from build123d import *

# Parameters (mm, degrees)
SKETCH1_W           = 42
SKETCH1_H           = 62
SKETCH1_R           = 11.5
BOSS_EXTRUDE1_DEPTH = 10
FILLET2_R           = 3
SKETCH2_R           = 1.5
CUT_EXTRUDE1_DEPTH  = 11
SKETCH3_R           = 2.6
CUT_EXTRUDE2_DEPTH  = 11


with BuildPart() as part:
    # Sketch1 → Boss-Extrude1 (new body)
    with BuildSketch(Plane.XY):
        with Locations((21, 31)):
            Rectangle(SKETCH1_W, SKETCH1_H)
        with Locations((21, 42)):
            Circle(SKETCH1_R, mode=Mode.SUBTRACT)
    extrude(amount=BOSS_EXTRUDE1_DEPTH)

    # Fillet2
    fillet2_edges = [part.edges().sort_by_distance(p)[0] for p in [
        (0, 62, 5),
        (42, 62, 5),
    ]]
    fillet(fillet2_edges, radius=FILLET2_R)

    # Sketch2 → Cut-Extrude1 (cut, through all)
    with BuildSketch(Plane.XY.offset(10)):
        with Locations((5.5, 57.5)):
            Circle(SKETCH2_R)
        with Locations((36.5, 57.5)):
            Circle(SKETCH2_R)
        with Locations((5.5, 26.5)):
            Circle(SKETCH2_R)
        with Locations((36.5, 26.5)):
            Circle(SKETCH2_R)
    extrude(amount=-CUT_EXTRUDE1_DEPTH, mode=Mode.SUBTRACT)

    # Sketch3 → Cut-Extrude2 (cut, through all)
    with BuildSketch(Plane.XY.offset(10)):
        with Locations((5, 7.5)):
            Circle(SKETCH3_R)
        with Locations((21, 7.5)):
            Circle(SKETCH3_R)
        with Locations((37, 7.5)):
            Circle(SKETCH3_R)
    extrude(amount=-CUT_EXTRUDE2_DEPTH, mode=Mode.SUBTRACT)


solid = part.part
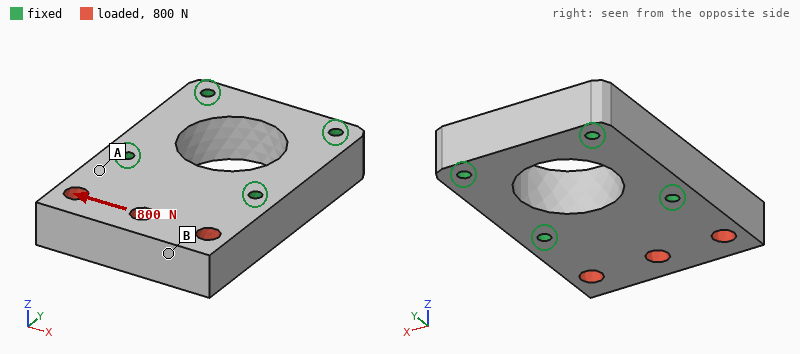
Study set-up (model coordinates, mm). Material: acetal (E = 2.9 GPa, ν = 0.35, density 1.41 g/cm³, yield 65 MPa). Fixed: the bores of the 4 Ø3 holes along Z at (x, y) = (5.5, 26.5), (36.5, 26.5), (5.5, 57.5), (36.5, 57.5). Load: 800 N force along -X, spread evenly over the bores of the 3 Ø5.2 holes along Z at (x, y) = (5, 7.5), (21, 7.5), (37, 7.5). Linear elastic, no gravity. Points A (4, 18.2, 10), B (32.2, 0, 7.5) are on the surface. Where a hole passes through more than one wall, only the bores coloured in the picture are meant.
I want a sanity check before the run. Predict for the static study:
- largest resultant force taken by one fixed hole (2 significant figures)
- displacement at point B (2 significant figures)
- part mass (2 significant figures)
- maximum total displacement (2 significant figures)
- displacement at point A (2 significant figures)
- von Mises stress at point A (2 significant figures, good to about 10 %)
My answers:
590 N
72 µm
30 g
74 µm
28 µm
2.9 MPa
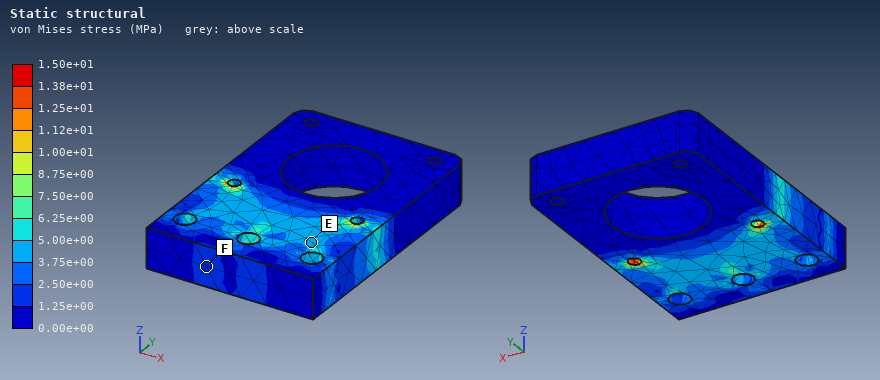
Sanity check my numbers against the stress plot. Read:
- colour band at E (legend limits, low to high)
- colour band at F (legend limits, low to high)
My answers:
3.75e+00 to 5.00e+00 MPa
1.25e+00 to 2.50e+00 MPa
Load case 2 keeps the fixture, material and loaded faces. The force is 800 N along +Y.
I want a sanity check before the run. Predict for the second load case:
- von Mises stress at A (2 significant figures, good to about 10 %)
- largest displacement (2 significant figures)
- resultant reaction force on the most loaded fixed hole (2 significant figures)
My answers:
2.7 MPa
23 µm
380 N
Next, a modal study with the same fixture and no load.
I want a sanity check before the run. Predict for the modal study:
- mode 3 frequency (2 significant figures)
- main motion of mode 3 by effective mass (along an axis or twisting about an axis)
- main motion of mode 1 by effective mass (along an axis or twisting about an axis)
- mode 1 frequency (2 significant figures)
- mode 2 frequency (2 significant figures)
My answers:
6200 Hz
along X
along Z
2500 Hz
4600 Hz
